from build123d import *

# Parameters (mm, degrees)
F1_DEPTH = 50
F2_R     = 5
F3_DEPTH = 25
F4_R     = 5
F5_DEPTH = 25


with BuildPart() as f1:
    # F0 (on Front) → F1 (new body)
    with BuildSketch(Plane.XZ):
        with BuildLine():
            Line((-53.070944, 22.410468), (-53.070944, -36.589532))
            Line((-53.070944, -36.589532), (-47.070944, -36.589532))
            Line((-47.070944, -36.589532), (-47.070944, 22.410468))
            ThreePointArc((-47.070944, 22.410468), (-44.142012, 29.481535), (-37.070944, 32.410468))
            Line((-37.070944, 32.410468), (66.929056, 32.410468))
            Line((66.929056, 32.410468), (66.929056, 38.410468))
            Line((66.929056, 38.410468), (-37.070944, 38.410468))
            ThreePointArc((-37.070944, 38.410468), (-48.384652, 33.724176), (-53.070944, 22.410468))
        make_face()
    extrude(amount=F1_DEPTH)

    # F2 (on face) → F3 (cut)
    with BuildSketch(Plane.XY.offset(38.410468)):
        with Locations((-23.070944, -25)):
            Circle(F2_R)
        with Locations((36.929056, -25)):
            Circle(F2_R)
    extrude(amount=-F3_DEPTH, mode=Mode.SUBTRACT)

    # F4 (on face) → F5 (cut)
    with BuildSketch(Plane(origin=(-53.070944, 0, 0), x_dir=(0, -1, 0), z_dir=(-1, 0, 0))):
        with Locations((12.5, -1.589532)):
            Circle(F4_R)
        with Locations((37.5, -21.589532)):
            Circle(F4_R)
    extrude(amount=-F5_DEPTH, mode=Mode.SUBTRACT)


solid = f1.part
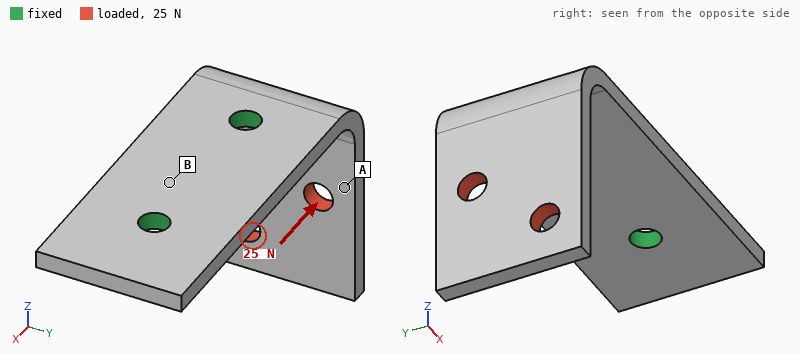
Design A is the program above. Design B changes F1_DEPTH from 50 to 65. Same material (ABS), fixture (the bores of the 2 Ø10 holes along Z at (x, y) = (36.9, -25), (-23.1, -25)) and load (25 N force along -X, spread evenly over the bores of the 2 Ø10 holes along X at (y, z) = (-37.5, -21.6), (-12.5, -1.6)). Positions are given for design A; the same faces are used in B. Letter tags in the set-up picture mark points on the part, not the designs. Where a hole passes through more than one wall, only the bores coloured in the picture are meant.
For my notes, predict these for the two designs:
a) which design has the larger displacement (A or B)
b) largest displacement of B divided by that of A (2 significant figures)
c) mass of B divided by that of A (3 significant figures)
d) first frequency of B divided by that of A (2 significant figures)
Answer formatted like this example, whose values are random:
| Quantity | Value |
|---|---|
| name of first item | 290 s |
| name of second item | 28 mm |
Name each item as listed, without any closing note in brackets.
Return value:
| Quantity | Value |
|---|---|
| which design has the larger displacement | A |
| largest displacement of B divided by that of A | 0.79 |
| mass of B divided by that of A | 1.31 |
| first frequency of B divided by that of A | 0.97 |
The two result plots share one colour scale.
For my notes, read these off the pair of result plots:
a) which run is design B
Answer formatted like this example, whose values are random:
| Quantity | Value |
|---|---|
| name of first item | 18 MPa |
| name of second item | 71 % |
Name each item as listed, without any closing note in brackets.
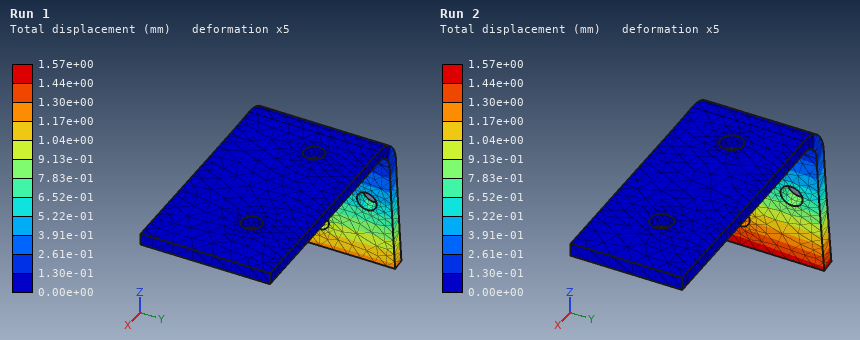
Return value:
| Quantity | Value |
|---|---|
| which run is design B | Run 1 |
